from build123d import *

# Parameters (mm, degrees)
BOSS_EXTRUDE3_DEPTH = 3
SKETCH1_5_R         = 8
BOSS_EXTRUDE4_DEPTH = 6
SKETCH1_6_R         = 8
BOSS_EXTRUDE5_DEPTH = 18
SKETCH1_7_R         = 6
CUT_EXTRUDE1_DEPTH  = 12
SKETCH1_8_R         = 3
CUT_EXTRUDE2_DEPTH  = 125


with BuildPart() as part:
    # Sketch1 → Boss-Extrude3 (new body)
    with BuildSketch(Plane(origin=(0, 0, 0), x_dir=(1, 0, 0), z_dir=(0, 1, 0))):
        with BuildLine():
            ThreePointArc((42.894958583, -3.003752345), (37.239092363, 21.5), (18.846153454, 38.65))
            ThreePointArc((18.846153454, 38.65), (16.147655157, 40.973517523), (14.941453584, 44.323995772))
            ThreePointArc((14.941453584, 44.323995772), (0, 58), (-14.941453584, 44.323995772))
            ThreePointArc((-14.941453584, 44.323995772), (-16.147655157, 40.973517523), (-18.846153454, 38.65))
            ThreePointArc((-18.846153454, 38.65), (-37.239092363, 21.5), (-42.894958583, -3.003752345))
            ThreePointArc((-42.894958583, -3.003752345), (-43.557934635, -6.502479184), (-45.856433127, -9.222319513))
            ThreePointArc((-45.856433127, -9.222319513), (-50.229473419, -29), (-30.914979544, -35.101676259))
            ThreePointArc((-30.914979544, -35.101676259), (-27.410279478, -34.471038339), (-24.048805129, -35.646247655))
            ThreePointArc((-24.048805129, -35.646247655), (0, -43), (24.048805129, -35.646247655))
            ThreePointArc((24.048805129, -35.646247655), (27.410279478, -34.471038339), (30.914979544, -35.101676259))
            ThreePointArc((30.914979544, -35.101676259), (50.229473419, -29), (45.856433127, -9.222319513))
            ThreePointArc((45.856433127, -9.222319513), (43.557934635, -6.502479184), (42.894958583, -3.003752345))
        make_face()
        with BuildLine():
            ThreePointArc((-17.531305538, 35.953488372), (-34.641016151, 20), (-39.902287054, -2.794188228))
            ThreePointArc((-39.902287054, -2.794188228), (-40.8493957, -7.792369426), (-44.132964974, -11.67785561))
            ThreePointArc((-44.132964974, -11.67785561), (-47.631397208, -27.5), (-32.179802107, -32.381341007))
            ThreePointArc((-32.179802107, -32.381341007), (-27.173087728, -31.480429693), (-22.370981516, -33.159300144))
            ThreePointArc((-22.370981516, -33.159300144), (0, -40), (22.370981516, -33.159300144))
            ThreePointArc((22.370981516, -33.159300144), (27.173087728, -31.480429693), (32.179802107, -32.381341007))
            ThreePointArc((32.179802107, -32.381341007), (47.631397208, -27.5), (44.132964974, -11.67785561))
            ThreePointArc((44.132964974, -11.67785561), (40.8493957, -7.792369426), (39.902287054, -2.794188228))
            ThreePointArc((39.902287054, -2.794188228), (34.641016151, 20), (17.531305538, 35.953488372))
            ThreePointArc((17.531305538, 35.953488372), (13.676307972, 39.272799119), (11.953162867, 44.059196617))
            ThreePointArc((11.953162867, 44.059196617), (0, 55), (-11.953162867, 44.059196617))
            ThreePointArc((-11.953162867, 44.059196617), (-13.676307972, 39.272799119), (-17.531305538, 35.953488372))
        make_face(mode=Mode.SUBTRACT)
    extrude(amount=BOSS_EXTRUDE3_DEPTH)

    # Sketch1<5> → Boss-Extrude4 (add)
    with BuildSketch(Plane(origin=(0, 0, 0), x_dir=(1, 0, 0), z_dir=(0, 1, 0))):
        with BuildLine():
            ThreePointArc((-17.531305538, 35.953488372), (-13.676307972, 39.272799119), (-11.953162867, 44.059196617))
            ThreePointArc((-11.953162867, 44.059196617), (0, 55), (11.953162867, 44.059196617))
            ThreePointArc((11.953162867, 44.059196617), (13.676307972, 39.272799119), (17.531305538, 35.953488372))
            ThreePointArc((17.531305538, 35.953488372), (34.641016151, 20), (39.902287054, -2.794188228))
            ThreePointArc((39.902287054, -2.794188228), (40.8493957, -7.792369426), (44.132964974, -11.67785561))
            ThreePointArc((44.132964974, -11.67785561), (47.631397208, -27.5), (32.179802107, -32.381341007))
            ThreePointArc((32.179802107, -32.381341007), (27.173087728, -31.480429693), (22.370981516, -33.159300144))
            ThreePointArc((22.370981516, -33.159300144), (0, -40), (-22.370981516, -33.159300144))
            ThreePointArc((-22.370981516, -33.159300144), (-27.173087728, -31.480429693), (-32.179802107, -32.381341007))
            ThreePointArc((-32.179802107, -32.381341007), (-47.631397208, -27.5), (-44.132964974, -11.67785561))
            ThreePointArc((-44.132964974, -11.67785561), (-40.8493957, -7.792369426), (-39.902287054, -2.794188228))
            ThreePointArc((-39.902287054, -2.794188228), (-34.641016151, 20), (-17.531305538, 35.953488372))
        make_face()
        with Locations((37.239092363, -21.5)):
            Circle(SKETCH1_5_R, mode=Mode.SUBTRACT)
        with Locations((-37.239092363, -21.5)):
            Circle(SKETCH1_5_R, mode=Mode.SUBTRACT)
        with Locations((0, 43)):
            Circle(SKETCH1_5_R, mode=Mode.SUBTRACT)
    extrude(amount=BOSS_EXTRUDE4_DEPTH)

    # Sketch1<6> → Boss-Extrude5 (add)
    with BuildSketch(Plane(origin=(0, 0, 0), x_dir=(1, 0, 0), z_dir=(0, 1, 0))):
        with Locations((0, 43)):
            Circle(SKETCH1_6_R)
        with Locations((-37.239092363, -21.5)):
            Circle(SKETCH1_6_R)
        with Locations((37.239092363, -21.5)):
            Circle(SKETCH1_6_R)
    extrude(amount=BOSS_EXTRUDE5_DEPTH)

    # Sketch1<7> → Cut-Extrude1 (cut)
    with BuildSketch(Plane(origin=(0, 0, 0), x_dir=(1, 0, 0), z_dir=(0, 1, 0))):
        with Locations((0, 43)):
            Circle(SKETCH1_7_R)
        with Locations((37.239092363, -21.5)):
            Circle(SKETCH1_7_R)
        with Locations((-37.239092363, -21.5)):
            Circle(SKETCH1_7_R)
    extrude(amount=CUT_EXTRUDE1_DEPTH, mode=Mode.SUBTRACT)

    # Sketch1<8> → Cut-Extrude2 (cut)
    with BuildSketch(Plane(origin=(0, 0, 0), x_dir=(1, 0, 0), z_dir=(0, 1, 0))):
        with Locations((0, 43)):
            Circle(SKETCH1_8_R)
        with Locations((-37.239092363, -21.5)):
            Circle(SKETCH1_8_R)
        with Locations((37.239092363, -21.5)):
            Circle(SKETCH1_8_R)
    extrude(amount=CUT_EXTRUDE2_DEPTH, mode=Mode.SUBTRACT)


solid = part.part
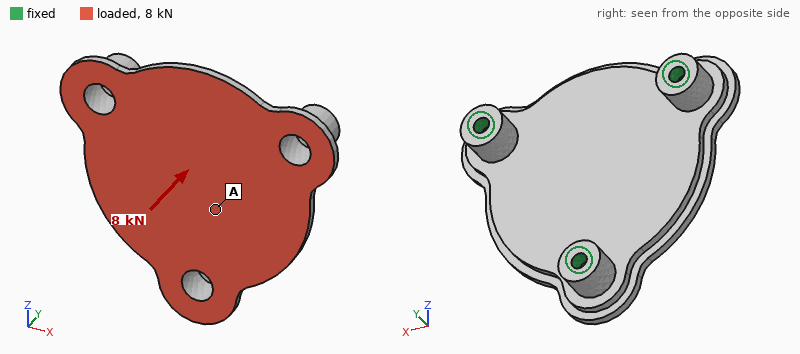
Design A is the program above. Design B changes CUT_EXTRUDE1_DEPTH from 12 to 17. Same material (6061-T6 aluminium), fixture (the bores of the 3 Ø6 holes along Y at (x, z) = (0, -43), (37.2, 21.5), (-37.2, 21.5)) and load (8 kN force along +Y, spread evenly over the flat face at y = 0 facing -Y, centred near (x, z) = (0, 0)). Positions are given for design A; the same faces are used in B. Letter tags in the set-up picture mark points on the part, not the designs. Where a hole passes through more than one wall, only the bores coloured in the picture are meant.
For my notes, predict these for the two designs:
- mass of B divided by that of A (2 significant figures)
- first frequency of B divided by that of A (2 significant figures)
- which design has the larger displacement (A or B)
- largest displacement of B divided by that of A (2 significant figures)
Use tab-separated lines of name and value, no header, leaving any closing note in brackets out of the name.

mass of B divided by that of A	0.97
first frequency of B divided by that of A	0.61
which design has the larger displacement	B
largest displacement of B divided by that of A	1.6
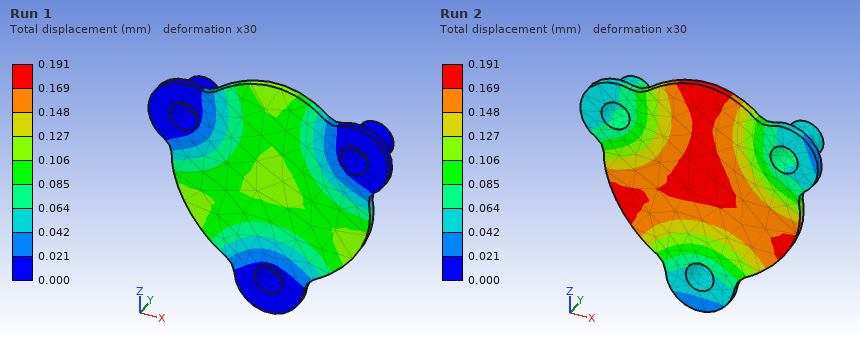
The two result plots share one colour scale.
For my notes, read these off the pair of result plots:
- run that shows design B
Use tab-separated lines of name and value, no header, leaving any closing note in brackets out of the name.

run that shows design B	Run 2
